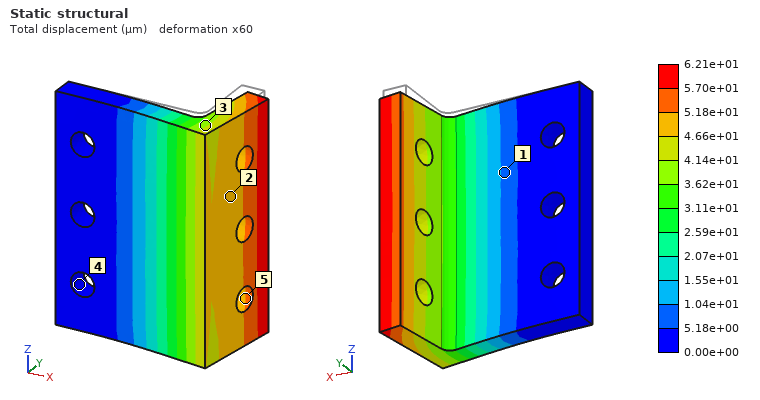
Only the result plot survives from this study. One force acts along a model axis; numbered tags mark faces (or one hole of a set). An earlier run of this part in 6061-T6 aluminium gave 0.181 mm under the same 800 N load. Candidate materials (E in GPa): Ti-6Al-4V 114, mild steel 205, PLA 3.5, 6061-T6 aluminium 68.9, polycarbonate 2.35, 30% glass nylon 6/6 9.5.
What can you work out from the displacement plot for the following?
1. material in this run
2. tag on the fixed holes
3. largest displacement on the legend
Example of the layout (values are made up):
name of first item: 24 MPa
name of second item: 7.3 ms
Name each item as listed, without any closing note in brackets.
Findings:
material in this run: mild steel
tag on the fixed holes: 4
largest displacement on the legend: 6.21e+01 µm
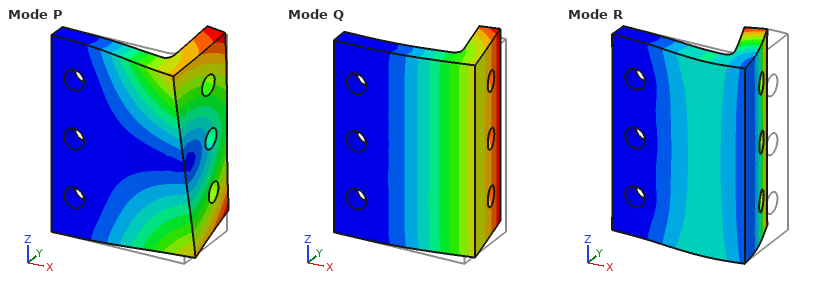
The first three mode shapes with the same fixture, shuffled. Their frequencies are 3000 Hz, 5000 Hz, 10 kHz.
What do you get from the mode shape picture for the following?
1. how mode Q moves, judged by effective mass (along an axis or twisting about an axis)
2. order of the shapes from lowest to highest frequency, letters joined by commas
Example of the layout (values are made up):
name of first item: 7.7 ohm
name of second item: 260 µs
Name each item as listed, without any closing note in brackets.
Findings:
how mode Q moves, judged by effective mass: along Y
order of the shapes from lowest to highest frequency, letters joined by commas: Q, P, R
